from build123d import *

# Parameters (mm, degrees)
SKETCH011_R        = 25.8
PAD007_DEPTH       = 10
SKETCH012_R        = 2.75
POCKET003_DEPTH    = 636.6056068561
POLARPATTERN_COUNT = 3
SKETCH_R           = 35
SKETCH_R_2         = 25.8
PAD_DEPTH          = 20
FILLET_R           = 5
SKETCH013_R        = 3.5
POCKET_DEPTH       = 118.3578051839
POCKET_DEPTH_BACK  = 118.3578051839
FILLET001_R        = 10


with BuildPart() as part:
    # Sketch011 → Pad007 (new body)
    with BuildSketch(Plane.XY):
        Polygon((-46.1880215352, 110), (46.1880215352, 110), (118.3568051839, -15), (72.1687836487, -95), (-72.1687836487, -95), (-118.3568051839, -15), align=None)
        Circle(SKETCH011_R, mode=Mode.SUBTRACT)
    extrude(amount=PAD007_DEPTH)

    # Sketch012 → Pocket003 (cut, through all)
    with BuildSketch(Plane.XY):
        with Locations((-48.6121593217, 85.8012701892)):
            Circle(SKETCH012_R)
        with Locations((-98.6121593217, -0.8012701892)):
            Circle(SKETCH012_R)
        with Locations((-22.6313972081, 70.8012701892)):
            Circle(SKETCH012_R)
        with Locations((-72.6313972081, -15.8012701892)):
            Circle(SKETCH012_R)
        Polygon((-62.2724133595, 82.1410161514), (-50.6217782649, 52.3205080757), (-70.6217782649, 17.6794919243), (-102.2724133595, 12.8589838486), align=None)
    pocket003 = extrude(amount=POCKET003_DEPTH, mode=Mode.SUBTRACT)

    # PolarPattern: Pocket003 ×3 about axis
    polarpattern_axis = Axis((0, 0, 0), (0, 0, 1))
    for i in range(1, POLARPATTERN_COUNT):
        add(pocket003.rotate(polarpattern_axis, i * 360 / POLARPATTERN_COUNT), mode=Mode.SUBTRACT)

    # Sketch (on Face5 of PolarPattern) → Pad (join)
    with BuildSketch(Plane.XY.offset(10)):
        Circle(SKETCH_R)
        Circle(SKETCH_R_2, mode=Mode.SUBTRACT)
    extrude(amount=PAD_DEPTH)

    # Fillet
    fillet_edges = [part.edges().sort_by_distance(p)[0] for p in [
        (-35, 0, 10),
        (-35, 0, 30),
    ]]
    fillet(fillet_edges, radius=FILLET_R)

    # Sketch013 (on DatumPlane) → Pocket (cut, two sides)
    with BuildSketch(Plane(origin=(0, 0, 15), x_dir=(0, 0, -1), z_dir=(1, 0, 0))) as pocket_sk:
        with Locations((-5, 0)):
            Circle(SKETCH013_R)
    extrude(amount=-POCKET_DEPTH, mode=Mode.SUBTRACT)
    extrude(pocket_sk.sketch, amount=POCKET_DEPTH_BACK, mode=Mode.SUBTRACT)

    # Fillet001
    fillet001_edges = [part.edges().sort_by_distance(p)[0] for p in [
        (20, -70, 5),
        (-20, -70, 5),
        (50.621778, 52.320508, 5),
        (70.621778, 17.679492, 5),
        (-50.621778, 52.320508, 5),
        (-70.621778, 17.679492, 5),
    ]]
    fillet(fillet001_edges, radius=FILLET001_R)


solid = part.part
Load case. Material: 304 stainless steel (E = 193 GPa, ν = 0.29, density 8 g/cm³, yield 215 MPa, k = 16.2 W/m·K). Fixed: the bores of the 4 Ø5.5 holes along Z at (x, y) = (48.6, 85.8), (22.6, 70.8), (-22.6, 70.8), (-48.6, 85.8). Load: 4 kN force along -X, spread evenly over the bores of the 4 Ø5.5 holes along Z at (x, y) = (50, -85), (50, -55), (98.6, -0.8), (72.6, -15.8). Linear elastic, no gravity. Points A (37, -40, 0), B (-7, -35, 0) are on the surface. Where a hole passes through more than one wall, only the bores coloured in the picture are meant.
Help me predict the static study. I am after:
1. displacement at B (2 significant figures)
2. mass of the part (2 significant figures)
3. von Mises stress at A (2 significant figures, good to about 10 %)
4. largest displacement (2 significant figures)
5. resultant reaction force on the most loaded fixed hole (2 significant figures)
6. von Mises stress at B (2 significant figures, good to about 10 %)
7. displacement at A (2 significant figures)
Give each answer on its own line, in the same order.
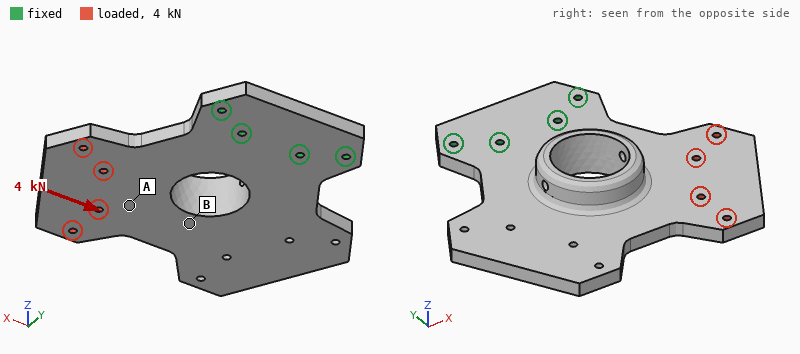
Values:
23 µm
2.6 kg
4.5 MPa
41 µm
3.4 kN
11 MPa
25 µm
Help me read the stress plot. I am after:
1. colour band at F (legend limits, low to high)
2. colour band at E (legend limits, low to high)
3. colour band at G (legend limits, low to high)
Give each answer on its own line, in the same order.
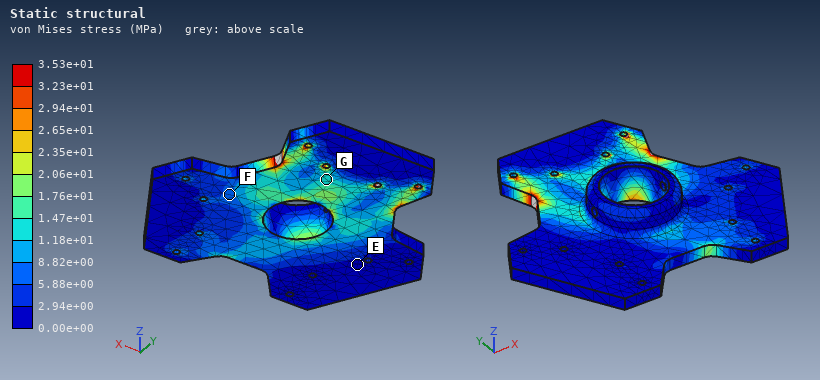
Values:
5.88e+00 to 8.82e+00 MPa
0.00e+00 to 2.94e+00 MPa
1.18e+01 to 1.47e+01 MPa
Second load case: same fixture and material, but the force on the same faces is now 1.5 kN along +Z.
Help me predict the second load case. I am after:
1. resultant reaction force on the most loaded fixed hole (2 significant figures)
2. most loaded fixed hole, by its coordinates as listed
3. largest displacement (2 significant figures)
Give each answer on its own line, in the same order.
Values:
3.1 kN
(22.6, 70.8)
0.76 mm
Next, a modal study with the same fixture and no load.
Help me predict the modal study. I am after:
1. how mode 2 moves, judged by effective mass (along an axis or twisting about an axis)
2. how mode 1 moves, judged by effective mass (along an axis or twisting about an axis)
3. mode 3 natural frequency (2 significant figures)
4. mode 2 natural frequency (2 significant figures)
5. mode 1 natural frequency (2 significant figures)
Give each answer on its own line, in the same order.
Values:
twisting about Y
along Z
1300 Hz
500 Hz
260 Hz
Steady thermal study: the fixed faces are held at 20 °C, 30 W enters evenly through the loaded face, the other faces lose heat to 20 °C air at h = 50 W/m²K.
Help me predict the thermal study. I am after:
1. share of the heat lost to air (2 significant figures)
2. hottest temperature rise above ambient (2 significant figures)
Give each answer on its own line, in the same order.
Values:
97 %
46 K
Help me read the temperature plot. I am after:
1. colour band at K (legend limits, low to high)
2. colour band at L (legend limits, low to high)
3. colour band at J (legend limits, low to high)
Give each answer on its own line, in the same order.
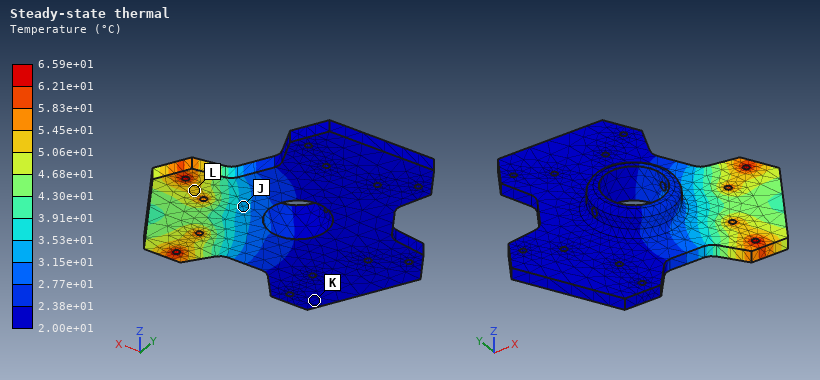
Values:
2.00e+01 to 2.38e+01 °C
5.06e+01 to 5.45e+01 °C
3.15e+01 to 3.53e+01 °C
